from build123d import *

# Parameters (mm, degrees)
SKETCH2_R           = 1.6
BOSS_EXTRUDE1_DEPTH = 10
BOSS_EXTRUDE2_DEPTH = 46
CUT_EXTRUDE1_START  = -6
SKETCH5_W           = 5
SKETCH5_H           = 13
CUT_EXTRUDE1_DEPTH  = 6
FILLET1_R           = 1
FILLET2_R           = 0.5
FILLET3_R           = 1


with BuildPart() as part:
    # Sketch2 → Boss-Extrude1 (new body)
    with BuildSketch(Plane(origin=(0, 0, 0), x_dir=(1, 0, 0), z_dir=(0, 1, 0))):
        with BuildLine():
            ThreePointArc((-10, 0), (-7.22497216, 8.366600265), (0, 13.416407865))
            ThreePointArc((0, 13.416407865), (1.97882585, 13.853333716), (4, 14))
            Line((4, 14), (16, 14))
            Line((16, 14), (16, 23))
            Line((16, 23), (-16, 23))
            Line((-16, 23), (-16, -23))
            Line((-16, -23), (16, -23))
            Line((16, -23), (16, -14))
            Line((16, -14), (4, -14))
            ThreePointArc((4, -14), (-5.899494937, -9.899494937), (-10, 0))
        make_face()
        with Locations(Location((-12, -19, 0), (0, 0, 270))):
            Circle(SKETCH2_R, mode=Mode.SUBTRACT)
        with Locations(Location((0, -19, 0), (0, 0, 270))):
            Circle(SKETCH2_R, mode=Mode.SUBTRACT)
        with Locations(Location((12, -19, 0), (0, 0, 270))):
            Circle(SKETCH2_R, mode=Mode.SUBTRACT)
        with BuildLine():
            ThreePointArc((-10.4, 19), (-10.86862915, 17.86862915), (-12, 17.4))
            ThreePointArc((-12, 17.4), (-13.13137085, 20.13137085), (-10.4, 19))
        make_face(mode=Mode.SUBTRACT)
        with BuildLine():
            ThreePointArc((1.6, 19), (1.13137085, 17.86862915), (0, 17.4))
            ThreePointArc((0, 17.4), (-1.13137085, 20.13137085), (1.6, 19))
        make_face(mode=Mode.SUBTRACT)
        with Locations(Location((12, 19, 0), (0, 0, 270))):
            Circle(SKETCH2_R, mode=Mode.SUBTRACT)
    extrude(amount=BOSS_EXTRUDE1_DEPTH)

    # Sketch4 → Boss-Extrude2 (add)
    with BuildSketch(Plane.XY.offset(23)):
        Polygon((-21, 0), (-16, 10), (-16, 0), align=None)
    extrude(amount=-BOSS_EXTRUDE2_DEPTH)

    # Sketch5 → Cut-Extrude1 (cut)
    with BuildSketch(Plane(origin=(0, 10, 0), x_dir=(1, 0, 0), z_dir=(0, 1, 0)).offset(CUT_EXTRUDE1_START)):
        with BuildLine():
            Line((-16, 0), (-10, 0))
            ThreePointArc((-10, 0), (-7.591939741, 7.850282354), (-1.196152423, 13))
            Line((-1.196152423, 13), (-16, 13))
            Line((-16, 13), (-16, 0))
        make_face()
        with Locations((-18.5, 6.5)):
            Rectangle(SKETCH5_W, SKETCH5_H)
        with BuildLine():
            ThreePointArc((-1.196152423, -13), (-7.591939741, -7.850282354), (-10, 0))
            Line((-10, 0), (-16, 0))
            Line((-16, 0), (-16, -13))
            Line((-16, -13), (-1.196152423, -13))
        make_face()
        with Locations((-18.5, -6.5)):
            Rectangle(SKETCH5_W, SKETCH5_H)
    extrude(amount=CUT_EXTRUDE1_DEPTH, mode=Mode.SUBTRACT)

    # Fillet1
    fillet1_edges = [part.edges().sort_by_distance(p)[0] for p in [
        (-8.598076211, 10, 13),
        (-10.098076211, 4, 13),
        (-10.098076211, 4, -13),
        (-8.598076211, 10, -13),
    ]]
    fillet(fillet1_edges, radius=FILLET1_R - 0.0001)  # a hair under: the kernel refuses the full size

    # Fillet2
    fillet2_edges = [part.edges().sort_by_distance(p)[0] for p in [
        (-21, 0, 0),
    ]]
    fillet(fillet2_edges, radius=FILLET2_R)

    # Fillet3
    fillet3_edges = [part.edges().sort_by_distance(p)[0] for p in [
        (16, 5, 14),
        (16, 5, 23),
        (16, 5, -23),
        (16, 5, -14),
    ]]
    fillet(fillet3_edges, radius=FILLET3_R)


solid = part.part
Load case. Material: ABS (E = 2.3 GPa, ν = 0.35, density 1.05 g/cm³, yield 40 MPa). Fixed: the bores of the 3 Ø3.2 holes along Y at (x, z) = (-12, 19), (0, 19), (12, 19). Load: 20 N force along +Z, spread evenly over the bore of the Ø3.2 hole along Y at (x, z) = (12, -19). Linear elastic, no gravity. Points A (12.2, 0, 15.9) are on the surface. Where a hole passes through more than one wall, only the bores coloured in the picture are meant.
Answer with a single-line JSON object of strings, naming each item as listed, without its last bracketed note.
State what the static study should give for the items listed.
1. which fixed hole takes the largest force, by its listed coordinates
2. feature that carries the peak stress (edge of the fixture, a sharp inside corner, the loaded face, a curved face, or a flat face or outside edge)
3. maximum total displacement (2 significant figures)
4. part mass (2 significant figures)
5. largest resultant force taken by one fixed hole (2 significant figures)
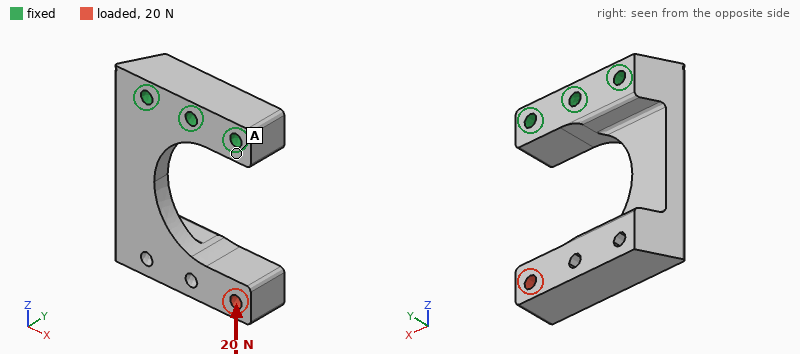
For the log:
{"which fixed hole takes the largest force, by its listed coordinates": "(0, 19)", "feature that carries the peak stress": "a curved face", "maximum total displacement": "0.69 mm", "part mass": "7.8 g", "largest resultant force taken by one fixed hole": "36 N"}
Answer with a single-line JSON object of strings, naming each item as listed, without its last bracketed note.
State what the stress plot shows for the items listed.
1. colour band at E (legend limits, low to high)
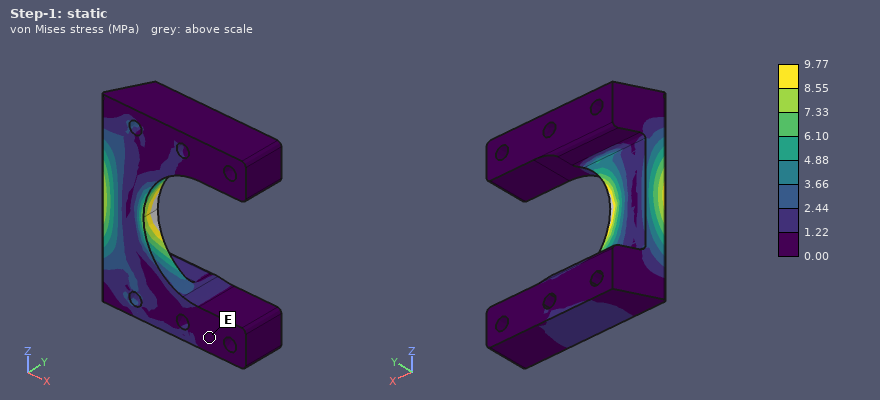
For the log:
{"colour band at E": "0.00 to 1.22 MPa"}
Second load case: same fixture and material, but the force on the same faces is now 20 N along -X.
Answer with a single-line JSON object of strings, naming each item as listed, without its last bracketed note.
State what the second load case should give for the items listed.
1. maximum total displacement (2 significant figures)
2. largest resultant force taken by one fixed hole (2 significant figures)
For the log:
{"maximum total displacement": "0.60 mm", "largest resultant force taken by one fixed hole": "54 N"}
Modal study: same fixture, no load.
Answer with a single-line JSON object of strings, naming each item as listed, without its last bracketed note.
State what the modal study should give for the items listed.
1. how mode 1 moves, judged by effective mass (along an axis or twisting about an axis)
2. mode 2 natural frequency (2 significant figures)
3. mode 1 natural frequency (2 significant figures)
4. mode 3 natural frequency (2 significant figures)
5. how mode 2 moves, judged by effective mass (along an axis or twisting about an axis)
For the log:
{"how mode 1 moves, judged by effective mass": "along Y", "mode 2 natural frequency": "600 Hz", "mode 1 natural frequency": "260 Hz", "mode 3 natural frequency": "770 Hz", "how mode 2 moves, judged by effective mass": "along X"}
